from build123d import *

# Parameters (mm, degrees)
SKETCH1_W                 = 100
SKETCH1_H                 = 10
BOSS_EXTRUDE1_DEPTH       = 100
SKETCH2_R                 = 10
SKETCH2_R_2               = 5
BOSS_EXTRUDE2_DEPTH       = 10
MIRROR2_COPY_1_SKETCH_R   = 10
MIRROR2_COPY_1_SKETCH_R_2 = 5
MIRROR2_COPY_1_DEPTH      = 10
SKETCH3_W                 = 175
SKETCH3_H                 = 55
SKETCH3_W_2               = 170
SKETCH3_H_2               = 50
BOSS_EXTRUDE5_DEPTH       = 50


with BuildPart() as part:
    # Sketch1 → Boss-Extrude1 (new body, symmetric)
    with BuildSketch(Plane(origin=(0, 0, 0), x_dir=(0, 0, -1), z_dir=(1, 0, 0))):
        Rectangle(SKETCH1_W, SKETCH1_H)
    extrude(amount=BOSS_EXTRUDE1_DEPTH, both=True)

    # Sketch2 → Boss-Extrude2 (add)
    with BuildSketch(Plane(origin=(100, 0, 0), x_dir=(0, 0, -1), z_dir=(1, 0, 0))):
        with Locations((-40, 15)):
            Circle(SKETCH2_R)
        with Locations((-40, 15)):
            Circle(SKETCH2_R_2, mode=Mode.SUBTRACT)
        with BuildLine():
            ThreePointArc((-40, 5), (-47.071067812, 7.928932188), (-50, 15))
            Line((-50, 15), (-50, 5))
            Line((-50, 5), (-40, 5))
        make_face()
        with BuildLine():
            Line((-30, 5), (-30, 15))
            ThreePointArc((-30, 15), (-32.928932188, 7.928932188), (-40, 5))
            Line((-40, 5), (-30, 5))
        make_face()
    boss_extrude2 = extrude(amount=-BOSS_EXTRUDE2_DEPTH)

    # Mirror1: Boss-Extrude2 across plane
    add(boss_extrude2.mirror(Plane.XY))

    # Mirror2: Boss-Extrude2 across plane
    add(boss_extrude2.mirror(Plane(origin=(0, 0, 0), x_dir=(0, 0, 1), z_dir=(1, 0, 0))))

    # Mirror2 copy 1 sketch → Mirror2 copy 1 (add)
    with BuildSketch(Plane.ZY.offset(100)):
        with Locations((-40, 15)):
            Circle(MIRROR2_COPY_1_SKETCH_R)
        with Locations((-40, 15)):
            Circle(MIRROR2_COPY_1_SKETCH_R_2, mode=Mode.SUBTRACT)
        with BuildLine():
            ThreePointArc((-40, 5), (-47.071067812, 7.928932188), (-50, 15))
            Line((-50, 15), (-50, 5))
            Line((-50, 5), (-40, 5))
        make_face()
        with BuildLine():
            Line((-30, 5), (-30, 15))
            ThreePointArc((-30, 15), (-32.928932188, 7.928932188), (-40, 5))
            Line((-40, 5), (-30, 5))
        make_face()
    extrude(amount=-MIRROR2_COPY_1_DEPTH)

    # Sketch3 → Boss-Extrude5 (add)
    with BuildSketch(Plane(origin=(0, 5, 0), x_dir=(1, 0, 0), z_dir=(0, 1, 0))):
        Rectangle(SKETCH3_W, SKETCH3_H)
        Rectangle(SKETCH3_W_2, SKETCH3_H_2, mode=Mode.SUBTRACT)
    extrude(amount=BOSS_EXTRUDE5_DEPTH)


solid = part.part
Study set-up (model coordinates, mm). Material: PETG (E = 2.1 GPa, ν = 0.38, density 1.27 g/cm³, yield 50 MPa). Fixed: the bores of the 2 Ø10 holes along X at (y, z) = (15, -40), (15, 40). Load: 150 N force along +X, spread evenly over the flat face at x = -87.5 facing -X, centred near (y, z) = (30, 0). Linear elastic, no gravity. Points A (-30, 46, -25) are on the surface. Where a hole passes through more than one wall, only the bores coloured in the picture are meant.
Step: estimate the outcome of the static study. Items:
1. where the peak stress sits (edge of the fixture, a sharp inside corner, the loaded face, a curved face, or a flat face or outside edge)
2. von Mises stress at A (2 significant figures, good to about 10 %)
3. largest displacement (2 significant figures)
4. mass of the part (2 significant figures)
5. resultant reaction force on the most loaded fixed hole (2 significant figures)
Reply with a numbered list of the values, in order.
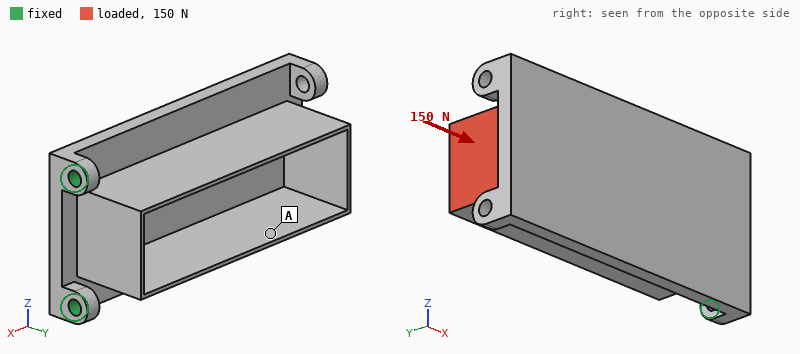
1. the loaded face
2. 0.93 MPa
3. 2.6 mm
4. 340 g
5. 75 N
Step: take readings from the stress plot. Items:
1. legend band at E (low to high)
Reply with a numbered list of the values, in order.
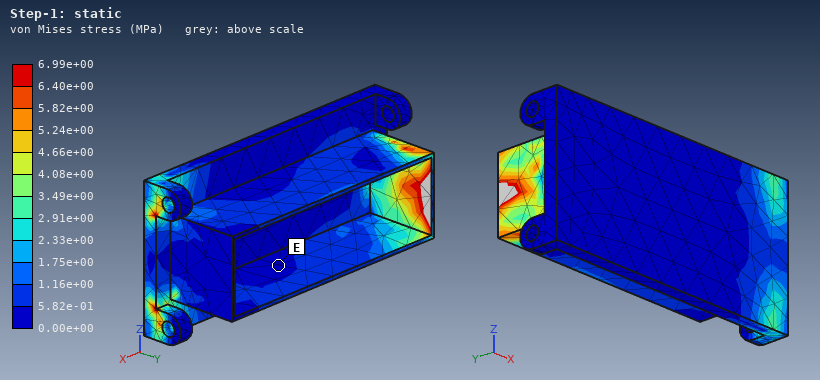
1. 0.00e+00 to 5.82e-01 MPa
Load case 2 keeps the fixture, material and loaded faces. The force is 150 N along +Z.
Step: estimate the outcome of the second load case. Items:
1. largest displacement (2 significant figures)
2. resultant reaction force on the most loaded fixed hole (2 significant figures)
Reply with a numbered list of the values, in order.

1. 2.5 mm
2. 340 N
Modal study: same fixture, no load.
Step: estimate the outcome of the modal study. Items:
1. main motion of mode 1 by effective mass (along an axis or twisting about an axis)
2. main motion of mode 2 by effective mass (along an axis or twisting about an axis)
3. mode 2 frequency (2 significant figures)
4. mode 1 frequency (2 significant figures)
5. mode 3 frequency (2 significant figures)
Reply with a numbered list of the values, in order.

1. along Y
2. along Z
3. 160 Hz
4. 46 Hz
5. 270 Hz
